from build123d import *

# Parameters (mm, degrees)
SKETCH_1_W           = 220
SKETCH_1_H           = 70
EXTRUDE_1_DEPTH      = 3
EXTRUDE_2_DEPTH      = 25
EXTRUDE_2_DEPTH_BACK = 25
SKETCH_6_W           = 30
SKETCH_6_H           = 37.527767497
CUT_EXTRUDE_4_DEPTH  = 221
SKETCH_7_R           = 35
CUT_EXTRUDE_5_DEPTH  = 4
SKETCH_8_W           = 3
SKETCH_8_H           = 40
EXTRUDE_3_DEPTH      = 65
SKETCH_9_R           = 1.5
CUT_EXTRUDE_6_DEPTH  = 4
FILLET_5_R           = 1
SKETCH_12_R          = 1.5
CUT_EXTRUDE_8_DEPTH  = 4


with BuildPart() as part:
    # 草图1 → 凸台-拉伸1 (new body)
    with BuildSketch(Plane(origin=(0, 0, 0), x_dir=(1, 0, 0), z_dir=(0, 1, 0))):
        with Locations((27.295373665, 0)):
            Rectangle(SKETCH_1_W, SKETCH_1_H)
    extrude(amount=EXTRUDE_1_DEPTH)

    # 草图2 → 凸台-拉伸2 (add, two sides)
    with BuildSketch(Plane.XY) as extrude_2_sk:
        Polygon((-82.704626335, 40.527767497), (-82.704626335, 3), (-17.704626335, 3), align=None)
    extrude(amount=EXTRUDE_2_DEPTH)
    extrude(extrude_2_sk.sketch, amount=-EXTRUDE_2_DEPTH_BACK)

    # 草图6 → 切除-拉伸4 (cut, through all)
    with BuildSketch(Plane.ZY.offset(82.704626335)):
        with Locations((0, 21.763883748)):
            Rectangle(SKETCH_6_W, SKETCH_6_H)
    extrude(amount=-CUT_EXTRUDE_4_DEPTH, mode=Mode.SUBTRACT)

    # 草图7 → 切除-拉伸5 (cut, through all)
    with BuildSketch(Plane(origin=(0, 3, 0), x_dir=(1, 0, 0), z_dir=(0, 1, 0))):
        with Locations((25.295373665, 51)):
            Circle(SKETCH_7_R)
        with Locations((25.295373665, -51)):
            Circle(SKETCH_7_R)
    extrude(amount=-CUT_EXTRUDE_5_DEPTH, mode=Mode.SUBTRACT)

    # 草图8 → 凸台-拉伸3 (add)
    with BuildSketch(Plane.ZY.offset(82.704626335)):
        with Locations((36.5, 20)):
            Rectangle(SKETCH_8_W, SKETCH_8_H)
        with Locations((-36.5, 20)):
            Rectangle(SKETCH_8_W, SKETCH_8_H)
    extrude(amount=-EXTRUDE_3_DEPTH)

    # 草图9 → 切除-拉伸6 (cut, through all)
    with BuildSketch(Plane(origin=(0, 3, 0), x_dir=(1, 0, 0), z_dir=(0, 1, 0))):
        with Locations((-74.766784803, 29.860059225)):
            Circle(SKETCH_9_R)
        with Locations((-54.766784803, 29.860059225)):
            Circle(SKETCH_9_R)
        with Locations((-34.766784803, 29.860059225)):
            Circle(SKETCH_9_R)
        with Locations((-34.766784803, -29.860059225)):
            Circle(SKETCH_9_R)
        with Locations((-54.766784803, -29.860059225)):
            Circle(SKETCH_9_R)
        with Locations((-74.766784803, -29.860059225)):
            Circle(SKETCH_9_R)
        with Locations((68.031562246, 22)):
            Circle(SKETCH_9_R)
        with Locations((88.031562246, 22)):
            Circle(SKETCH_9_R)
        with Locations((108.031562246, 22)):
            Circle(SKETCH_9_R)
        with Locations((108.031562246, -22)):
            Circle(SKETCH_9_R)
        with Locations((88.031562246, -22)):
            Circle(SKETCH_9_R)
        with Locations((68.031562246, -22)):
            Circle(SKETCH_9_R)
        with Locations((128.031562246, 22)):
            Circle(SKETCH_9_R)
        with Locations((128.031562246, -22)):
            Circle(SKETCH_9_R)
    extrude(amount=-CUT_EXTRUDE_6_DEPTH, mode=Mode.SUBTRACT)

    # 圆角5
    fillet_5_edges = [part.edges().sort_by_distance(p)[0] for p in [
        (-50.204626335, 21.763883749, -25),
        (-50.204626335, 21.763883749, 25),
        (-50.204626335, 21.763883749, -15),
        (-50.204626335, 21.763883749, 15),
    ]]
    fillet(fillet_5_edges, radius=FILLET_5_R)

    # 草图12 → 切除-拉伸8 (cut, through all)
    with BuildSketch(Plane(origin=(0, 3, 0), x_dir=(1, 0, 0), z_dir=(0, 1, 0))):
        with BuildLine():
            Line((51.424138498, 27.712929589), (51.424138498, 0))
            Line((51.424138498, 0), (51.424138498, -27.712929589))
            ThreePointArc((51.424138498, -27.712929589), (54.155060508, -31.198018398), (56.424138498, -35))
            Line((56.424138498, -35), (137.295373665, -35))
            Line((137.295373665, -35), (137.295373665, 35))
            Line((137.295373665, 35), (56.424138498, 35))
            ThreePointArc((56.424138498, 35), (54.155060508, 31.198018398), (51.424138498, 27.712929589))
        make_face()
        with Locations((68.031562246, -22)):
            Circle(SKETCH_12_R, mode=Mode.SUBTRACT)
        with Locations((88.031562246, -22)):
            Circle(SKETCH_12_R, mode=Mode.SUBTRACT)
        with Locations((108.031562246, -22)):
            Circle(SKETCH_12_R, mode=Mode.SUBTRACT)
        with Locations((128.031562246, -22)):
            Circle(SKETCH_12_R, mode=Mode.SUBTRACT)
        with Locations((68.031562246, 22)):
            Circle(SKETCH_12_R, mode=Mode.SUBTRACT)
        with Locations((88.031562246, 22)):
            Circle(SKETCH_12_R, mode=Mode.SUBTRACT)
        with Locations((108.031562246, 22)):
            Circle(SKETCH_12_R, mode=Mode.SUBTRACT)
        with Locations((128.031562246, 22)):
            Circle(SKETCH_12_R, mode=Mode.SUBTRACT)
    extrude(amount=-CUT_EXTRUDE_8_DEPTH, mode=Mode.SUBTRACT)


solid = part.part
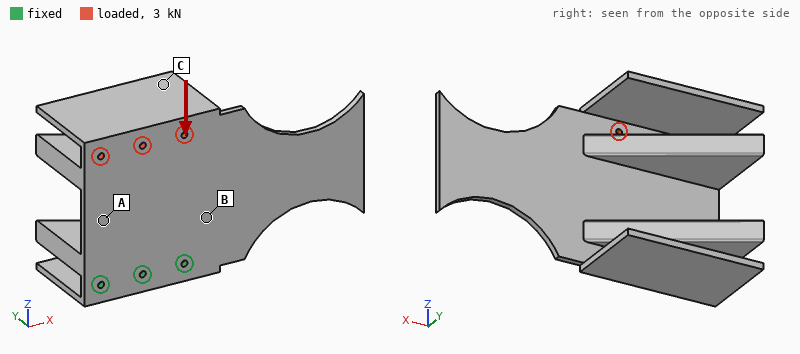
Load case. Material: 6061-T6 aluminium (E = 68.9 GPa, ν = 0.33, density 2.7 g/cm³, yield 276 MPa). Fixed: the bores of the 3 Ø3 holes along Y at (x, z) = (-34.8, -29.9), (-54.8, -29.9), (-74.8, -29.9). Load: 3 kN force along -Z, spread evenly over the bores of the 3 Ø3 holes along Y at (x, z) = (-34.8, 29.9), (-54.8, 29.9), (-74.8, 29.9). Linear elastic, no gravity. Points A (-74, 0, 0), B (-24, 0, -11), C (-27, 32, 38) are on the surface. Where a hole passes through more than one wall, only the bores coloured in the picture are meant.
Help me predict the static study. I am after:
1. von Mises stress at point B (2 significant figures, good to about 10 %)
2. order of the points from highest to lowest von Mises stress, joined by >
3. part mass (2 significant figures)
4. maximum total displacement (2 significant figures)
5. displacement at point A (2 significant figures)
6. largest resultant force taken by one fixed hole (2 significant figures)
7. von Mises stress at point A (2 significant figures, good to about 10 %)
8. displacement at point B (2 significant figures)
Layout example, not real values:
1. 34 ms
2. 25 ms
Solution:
1. 8.1 MPa
2. A > B > C
3. 170 g
4. 34 µm
5. 12 µm
6. 1.0 kN
7. 18 MPa
8. 6.3 µm
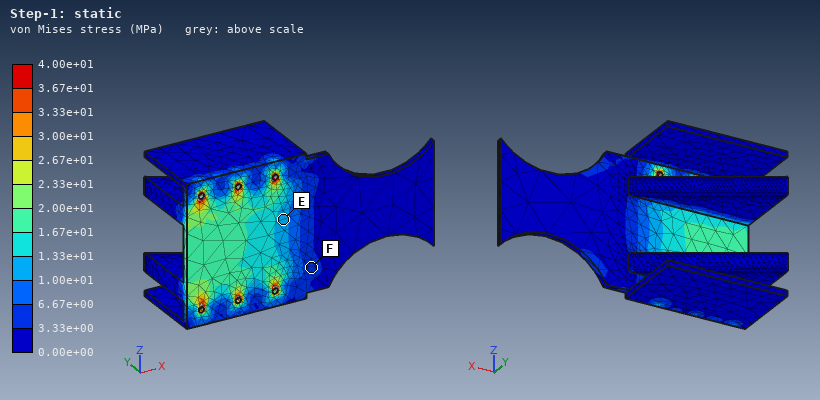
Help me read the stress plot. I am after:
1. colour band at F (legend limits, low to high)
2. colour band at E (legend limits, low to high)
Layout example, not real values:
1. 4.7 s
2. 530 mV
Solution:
1. 3.33e+00 to 6.67e+00 MPa
2. 1.00e+01 to 1.33e+01 MPa
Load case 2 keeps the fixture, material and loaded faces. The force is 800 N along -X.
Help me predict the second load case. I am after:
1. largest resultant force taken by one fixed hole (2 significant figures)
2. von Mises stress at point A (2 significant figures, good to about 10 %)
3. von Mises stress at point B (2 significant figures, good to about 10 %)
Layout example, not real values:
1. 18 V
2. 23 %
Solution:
1. 1.2 kN
2. 11 MPa
3. 7.4 MPa
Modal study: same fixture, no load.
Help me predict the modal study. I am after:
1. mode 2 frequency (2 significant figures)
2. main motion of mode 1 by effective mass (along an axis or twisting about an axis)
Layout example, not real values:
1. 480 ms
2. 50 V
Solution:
1. 460 Hz
2. along Y
